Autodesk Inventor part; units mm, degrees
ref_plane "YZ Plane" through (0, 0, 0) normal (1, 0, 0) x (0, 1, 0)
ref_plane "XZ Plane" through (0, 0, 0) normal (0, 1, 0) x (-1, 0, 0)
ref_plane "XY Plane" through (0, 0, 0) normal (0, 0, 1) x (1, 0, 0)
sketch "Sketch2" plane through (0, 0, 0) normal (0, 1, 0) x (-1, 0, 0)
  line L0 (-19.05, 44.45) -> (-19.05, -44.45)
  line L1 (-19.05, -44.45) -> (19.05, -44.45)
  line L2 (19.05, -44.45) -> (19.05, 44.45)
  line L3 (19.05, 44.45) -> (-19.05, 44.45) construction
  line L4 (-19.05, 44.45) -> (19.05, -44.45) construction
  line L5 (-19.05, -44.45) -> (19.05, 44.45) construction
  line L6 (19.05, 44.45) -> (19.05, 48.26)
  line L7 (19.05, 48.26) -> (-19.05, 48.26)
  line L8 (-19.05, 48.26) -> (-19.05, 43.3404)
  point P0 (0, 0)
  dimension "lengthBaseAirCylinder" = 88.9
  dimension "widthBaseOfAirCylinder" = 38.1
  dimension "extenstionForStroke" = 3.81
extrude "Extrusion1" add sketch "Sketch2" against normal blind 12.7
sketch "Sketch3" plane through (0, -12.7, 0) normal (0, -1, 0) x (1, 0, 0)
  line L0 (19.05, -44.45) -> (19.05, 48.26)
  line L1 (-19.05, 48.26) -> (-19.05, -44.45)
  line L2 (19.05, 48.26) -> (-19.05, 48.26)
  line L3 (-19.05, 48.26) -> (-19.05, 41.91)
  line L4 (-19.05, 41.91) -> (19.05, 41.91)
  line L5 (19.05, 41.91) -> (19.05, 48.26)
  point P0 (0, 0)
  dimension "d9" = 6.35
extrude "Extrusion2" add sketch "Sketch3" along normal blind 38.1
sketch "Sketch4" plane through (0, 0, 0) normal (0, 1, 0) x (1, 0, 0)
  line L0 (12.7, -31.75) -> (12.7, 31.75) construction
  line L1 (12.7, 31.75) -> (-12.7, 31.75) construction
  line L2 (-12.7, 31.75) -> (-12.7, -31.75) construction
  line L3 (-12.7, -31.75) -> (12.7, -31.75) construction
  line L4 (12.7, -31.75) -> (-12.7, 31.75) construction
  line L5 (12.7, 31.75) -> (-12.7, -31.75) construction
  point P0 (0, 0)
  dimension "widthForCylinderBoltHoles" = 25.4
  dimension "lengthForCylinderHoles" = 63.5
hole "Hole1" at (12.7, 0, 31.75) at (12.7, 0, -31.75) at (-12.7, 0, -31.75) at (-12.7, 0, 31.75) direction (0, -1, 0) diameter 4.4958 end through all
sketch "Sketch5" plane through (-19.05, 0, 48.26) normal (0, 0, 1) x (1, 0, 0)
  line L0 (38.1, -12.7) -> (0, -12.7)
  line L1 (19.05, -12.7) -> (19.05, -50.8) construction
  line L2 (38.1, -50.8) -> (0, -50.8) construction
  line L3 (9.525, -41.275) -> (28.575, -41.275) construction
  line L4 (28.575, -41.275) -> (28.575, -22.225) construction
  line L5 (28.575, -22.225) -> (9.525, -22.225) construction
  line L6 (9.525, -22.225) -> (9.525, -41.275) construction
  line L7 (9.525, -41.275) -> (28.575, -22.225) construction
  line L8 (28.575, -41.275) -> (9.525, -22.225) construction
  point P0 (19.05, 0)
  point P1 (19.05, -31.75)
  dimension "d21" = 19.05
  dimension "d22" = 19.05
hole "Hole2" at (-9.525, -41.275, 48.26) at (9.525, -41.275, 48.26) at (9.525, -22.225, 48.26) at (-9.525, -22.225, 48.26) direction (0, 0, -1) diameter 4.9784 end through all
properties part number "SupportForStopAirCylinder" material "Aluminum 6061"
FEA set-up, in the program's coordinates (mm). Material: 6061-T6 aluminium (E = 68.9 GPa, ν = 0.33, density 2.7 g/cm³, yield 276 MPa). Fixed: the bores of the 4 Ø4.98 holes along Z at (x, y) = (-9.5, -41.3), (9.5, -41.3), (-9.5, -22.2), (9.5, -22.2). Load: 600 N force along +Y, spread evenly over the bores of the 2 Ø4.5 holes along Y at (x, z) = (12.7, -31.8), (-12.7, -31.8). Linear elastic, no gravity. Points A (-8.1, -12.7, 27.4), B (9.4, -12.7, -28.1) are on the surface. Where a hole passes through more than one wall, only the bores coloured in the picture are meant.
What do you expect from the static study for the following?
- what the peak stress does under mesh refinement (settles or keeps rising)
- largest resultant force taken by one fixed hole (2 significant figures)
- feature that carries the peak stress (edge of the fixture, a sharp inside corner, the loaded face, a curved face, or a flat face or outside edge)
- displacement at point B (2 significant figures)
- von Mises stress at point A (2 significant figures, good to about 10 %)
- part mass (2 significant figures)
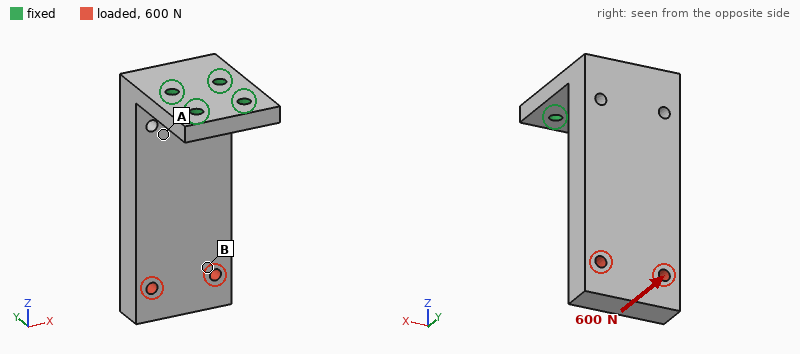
keeps rising
420 N
edge of the fixture
0.88 mm
41 MPa
140 g
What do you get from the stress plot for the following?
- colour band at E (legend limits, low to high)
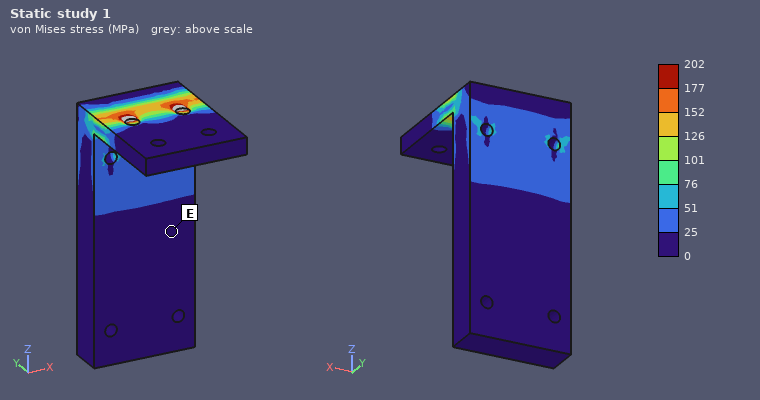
0 to 25 MPa
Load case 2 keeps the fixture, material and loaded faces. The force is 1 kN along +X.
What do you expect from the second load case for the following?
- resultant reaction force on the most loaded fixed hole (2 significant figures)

3.3 kN
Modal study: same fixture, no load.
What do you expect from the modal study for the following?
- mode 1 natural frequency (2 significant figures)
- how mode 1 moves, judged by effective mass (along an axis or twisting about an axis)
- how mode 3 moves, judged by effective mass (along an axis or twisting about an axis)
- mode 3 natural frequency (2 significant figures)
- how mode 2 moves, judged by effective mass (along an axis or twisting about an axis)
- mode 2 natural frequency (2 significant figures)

560 Hz
along Y
along Z
4400 Hz
along X
1300 Hz
